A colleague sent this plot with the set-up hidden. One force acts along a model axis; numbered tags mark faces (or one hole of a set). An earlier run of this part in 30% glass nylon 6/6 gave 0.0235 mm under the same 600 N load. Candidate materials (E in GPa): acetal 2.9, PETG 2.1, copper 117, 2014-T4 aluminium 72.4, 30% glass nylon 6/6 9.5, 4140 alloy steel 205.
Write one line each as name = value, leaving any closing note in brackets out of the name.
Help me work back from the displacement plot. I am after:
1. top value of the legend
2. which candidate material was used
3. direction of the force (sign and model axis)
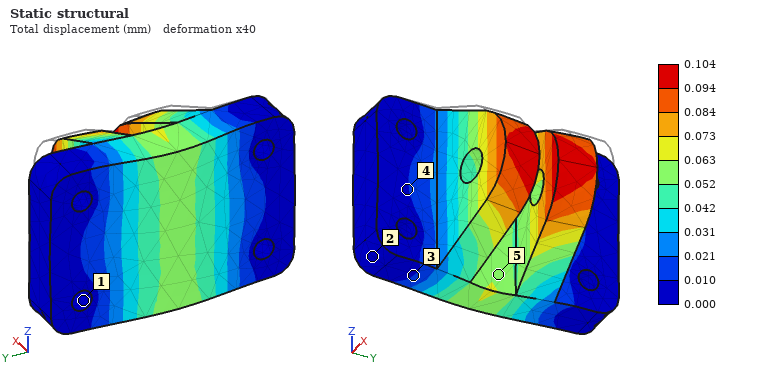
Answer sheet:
top value of the legend = 0.104 mm
which candidate material was used = PETG
direction of the force = -X
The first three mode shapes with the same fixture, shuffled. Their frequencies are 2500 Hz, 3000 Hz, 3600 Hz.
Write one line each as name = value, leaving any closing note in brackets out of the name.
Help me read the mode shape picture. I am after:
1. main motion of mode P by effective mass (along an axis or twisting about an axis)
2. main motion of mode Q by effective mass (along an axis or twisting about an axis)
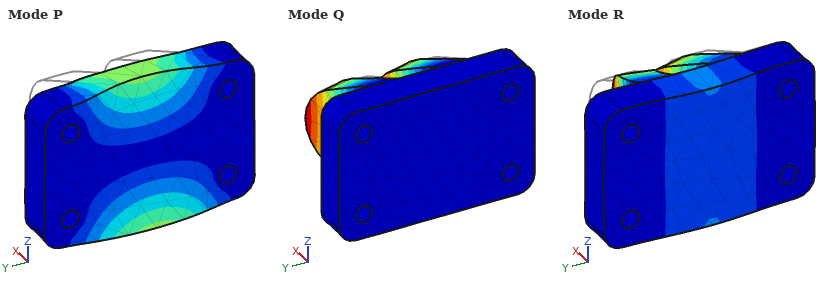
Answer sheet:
main motion of mode P by effective mass = along Z
main motion of mode Q by effective mass = along Y
